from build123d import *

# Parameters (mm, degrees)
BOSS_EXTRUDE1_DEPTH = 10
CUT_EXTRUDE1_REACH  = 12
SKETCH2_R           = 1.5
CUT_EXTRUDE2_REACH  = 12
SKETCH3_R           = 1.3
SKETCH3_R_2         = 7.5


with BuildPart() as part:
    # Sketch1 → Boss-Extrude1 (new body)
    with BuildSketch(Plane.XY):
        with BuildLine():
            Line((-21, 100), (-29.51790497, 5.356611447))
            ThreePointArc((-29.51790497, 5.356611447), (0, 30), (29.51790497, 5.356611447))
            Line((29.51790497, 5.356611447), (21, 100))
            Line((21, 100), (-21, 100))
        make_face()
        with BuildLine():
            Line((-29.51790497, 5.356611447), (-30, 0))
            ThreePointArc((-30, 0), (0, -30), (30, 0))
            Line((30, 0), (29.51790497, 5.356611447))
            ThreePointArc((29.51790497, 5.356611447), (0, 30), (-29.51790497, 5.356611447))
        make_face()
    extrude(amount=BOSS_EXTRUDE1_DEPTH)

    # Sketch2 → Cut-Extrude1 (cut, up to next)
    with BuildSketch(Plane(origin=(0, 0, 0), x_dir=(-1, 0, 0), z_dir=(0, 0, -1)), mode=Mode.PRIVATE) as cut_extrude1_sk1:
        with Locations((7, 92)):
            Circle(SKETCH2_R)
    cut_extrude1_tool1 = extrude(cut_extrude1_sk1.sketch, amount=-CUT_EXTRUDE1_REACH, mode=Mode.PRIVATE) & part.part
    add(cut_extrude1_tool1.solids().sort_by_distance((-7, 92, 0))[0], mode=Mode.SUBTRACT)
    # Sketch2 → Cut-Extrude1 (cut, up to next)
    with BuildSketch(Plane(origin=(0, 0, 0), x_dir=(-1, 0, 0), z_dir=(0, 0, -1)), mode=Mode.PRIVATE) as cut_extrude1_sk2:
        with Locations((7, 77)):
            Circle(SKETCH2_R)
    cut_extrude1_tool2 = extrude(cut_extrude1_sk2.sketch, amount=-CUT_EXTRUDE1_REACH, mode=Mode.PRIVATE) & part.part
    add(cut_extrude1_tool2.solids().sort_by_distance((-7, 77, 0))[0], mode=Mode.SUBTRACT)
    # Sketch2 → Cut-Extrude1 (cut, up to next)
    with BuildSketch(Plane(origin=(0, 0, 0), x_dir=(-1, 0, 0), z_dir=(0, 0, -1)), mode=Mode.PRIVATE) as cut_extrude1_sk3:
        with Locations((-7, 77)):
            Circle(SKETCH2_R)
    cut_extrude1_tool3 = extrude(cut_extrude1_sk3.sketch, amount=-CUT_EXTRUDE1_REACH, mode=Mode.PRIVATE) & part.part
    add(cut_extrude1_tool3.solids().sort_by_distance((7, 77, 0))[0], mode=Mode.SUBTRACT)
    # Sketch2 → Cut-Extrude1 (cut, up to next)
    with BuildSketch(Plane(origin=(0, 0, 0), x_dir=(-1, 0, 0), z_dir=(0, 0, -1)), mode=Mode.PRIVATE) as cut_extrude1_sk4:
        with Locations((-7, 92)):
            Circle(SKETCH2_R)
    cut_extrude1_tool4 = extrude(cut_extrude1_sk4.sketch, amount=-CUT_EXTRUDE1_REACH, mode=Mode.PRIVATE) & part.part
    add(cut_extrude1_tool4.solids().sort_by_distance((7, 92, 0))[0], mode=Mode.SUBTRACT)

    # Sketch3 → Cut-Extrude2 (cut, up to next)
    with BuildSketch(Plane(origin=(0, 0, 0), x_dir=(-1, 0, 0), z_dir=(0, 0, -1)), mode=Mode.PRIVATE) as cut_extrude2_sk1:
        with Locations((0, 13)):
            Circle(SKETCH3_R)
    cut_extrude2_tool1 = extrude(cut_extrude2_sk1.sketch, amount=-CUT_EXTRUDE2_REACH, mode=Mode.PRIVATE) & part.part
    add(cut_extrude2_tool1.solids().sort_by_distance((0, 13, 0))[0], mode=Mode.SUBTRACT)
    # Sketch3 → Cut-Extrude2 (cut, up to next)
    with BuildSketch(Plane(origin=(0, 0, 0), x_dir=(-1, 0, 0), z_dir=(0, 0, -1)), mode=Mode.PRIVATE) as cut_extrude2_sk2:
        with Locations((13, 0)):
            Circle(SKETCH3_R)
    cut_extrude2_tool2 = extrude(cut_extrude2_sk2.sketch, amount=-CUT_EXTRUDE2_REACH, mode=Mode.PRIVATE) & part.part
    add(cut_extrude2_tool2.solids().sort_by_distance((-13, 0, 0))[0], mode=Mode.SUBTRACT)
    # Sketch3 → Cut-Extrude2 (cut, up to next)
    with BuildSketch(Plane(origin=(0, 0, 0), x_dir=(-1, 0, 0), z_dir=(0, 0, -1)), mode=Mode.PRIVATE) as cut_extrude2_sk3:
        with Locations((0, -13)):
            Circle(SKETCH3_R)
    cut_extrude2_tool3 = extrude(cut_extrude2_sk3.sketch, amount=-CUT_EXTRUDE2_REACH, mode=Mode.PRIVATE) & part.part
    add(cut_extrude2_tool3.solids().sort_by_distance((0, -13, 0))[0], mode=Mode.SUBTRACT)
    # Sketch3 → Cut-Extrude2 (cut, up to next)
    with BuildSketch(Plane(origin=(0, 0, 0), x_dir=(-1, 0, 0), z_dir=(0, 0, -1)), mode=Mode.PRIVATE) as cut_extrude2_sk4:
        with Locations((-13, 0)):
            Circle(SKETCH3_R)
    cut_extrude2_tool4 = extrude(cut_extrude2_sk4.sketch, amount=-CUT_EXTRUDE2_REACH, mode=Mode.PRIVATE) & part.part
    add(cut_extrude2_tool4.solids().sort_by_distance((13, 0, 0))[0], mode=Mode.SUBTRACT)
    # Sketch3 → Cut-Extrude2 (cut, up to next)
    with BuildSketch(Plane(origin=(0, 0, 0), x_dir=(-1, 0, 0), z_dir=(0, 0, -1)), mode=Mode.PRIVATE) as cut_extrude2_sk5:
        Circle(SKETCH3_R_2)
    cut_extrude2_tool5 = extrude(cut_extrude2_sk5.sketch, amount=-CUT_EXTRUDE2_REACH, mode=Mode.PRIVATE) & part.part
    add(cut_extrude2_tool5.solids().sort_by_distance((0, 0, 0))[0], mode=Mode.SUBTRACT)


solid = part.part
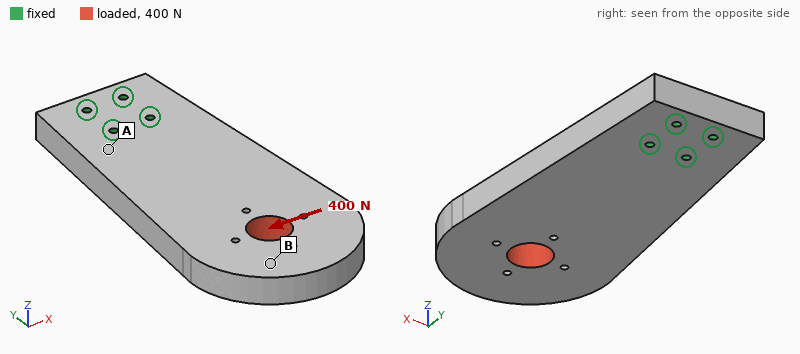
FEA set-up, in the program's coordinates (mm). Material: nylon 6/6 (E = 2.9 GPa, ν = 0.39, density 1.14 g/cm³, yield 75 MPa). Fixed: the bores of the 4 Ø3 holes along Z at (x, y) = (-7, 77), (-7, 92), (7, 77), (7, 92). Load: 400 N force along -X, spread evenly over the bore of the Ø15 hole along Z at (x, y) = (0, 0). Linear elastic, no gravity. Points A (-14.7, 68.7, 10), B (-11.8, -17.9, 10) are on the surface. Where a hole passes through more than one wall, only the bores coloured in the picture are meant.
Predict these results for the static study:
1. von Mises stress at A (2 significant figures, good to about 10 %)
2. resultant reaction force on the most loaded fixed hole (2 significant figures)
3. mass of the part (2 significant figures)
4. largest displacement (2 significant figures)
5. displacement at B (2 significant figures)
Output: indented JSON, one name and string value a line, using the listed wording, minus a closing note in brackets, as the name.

{
  "von Mises stress at A": "4.2 MPa",
  "resultant reaction force on the most loaded fixed hole": "1.0 kN",
  "mass of the part": "72 g",
  "largest displacement": "0.68 mm",
  "displacement at B": "0.61 mm"
}
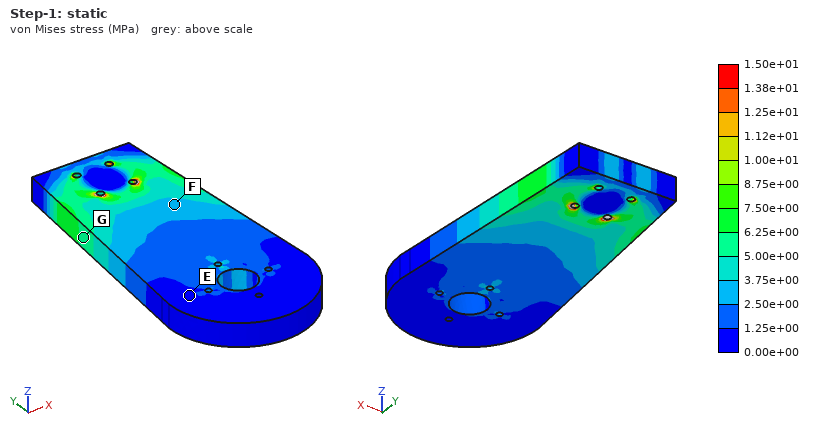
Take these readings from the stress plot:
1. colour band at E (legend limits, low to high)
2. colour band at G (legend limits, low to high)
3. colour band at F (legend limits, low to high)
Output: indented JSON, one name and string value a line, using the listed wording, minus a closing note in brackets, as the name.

{
  "colour band at E": "0.00e+00 to 1.25e+00 MPa",
  "colour band at G": "5.00e+00 to 6.25e+00 MPa",
  "colour band at F": "2.50e+00 to 3.75e+00 MPa"
}
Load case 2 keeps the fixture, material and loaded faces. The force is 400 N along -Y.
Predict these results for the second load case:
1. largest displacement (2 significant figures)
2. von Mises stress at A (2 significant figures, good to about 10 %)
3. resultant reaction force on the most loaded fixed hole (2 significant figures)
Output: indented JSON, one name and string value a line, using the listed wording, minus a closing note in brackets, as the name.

{
  "largest displacement": "31 µm",
  "von Mises stress at A": "0.74 MPa",
  "resultant reaction force on the most loaded fixed hole": "150 N"
}
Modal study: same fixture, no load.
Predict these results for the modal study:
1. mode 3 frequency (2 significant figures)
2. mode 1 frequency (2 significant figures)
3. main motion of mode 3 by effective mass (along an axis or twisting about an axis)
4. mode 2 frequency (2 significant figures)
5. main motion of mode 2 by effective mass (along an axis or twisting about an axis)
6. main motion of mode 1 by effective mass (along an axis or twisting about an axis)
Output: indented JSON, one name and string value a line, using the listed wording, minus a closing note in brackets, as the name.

{
  "mode 3 frequency": "790 Hz",
  "mode 1 frequency": "230 Hz",
  "main motion of mode 3 by effective mass": "twisting about Y",
  "mode 2 frequency": "750 Hz",
  "main motion of mode 2 by effective mass": "along X",
  "main motion of mode 1 by effective mass": "along Z"
}
